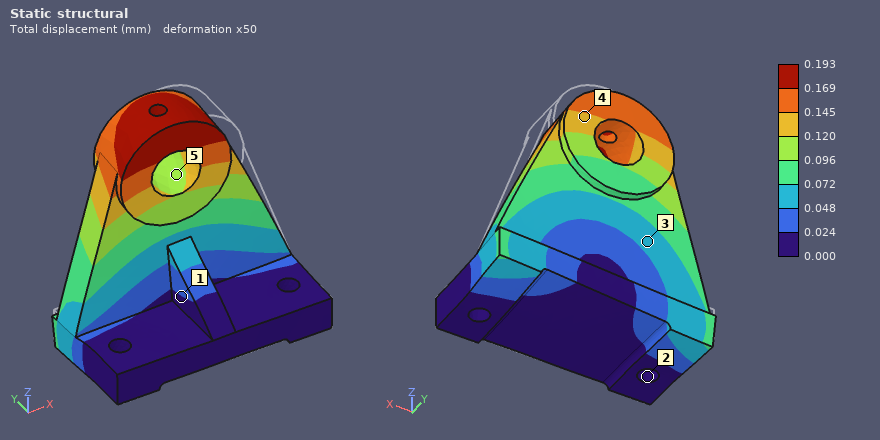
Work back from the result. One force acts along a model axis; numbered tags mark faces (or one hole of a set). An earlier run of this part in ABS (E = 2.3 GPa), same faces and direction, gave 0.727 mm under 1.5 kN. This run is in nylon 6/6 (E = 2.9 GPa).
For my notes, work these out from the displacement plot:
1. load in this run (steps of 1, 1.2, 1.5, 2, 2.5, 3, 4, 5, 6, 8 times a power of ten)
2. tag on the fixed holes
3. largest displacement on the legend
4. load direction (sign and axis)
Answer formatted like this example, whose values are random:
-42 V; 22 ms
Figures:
500 N; 2; 0.193 mm; -X
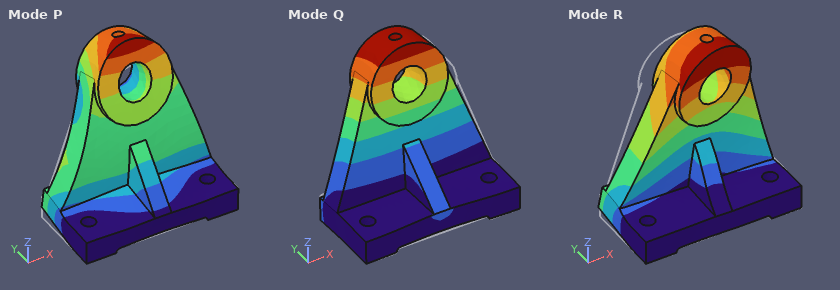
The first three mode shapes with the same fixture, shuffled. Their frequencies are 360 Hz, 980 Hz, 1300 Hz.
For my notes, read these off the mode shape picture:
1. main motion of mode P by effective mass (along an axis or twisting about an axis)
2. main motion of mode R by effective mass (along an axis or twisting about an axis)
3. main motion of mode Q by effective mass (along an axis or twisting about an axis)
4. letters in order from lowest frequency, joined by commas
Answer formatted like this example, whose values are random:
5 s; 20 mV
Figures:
along Z; along X; along Y; Q, R, P
